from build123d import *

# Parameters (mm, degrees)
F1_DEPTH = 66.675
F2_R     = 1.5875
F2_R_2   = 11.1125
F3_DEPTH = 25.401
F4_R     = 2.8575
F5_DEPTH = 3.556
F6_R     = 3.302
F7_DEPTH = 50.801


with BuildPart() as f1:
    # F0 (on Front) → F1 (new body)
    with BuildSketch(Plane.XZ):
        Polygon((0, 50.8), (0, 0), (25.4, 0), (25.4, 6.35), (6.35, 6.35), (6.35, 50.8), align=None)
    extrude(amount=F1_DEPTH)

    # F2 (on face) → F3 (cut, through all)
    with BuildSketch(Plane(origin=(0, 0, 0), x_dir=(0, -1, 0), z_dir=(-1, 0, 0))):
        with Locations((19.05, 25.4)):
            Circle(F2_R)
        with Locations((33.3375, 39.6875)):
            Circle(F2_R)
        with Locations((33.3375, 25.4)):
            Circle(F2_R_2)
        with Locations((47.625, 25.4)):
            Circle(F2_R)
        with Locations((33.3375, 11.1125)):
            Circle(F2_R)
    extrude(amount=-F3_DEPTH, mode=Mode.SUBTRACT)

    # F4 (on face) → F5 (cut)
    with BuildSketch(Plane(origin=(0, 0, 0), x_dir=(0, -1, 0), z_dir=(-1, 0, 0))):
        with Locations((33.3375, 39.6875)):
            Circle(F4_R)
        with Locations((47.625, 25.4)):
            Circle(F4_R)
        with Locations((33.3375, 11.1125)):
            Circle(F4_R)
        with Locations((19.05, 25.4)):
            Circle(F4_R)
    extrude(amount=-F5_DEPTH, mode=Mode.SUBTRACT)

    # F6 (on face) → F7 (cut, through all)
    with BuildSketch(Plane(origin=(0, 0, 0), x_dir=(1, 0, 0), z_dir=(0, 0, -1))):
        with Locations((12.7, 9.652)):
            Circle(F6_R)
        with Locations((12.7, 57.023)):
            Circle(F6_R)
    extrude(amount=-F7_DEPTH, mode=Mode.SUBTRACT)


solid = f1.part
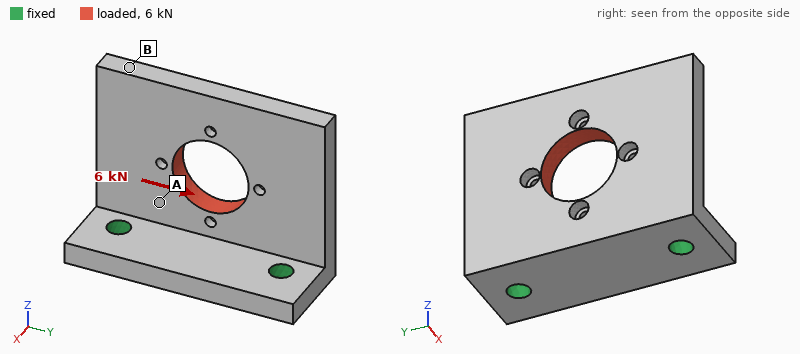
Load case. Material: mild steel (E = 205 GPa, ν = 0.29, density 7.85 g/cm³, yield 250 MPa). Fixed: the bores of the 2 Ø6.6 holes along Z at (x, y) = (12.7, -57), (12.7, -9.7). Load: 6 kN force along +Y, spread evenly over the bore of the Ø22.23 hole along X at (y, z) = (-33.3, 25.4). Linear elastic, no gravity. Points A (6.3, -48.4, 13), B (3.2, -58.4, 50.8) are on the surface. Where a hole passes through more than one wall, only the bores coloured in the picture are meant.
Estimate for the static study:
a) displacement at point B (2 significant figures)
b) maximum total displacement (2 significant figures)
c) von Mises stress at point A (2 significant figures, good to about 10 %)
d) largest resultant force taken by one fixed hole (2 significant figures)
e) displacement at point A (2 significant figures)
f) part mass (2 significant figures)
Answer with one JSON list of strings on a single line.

["30 µm", "33 µm", "43 MPa", "4.1 kN", "7.6 µm", "210 g"]
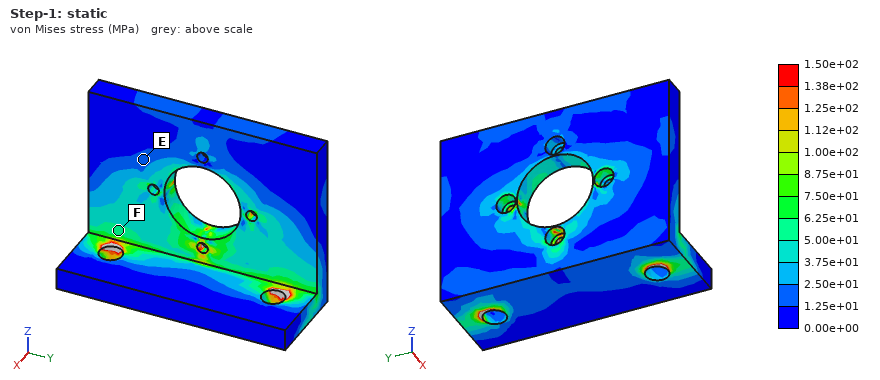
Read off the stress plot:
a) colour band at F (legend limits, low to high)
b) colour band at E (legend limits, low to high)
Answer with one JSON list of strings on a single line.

["5.00e+01 to 6.25e+01 MPa", "1.25e+01 to 2.50e+01 MPa"]
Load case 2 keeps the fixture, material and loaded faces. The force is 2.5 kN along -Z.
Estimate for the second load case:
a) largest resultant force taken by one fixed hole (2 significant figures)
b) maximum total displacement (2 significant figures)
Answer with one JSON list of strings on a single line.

["1.3 kN", "24 µm"]
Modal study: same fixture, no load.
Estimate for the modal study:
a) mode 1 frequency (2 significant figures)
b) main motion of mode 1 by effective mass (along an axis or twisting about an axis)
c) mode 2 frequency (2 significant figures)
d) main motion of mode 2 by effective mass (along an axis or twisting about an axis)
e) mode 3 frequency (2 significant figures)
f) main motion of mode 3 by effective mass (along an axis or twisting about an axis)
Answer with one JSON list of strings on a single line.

["1700 Hz", "along X", "3500 Hz", "twisting about Z", "6900 Hz", "along Y"]
